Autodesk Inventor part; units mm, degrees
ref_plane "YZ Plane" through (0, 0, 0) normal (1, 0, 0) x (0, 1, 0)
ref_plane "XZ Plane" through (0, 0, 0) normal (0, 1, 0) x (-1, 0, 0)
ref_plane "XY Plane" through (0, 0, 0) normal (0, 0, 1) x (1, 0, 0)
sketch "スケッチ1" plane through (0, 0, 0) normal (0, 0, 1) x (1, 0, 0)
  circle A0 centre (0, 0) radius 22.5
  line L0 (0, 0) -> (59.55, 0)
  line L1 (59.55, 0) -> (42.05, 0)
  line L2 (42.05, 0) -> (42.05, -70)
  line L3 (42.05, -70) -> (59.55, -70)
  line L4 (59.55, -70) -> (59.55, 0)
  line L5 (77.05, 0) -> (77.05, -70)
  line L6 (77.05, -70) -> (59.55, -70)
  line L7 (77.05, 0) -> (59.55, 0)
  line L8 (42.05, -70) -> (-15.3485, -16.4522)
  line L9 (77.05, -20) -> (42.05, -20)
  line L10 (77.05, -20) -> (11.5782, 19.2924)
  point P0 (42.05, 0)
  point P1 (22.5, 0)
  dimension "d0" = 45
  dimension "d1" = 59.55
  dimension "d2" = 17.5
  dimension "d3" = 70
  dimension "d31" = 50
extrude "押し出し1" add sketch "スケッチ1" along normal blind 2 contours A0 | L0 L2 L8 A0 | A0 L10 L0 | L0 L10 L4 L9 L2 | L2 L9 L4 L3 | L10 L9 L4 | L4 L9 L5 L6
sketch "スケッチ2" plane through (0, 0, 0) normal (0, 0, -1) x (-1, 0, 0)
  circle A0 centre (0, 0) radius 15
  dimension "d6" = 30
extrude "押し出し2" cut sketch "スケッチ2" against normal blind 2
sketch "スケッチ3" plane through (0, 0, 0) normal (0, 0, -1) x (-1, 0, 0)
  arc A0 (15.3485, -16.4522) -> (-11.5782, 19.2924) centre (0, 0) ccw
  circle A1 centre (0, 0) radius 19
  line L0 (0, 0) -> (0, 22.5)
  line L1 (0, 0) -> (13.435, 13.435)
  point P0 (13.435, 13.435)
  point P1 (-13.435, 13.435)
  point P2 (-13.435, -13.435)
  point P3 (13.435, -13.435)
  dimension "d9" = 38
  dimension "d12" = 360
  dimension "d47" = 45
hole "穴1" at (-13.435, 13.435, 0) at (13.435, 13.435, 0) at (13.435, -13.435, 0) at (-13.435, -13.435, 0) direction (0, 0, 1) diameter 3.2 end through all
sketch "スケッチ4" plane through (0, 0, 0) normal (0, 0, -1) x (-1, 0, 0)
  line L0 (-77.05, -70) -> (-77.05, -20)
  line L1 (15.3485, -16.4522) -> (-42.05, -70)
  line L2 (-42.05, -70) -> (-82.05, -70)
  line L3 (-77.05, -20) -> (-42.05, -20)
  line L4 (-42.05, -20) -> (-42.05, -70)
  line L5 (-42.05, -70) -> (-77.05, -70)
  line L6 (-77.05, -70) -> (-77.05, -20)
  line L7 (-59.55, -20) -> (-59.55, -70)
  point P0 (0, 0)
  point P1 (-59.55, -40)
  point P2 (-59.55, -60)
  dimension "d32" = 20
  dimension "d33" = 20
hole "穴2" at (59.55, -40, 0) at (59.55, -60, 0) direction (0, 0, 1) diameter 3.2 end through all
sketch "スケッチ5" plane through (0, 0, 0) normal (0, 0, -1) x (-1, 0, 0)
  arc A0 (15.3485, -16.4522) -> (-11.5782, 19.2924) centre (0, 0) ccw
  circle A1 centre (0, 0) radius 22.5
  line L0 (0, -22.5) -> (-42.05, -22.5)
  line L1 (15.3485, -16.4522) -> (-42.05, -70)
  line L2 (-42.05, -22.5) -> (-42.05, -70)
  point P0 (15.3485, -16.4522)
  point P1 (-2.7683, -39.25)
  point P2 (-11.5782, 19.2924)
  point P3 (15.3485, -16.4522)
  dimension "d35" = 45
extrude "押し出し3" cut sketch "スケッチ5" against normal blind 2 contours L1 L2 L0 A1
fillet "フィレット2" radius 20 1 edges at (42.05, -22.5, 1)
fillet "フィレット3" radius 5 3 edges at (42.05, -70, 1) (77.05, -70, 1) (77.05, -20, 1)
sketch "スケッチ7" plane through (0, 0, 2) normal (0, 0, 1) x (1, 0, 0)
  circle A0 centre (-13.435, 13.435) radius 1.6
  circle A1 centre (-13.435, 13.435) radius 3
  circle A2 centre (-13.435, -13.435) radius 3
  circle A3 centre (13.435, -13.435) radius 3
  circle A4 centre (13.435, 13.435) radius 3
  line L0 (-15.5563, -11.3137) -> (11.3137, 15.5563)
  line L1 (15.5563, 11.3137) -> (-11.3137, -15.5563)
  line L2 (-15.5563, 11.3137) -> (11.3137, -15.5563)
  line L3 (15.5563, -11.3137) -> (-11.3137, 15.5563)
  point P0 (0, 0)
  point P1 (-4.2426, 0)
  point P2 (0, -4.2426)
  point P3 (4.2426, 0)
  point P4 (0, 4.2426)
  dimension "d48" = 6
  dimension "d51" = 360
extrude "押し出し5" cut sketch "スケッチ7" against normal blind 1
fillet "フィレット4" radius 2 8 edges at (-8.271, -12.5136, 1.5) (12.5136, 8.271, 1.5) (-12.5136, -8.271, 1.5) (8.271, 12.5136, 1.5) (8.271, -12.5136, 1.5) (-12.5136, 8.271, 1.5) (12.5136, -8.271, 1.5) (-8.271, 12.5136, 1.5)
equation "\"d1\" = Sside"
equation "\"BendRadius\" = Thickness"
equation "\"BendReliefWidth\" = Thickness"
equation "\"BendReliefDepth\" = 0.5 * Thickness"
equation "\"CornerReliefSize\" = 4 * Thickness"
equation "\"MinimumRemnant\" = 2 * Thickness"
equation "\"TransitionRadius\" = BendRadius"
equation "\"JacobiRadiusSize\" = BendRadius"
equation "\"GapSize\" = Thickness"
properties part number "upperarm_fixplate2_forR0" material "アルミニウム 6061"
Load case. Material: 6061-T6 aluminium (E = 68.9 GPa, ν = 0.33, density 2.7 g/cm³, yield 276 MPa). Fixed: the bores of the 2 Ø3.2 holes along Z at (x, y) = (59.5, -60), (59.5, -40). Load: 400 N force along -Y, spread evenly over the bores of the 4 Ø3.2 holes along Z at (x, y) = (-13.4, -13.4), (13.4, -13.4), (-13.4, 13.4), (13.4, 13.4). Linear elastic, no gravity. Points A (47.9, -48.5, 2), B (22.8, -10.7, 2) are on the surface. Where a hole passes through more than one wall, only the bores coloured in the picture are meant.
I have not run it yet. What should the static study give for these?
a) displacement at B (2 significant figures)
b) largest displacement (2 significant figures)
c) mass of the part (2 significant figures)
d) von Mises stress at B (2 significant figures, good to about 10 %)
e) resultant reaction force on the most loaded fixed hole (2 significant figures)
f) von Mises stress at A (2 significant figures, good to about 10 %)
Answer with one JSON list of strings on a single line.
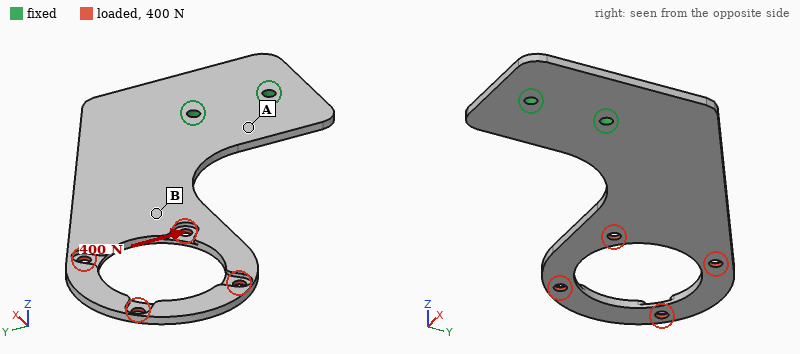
["0.15 mm", "0.50 mm", "20 g", "20 MPa", "1.1 kN", "40 MPa"]
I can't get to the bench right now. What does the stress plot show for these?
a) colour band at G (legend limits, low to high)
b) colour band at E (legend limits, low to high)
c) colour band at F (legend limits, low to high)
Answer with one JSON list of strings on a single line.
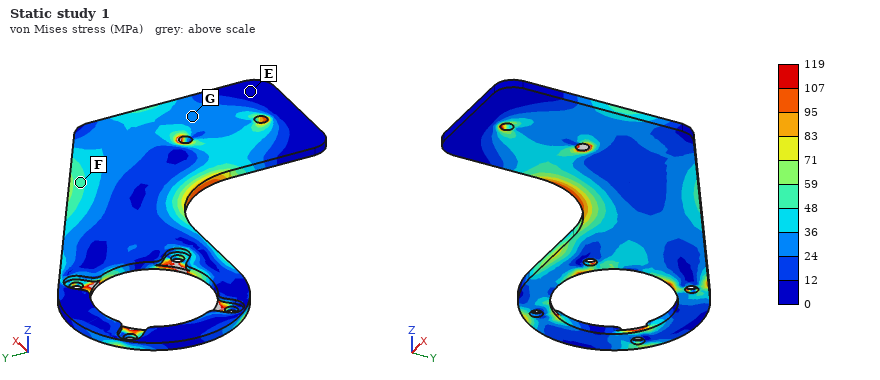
["24 to 36 MPa", "0 to 12 MPa", "48 to 59 MPa"]
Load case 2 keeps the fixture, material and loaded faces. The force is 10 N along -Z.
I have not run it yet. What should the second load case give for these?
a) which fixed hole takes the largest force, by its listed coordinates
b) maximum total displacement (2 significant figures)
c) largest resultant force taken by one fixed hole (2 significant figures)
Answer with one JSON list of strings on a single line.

["(59.5, -40)", "1.4 mm", "19 N"]
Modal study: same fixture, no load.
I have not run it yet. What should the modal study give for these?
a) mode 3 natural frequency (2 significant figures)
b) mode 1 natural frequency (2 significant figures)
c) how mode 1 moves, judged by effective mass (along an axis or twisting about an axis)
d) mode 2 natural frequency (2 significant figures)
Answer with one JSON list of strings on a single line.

["1000 Hz", "220 Hz", "along Z", "720 Hz"]
